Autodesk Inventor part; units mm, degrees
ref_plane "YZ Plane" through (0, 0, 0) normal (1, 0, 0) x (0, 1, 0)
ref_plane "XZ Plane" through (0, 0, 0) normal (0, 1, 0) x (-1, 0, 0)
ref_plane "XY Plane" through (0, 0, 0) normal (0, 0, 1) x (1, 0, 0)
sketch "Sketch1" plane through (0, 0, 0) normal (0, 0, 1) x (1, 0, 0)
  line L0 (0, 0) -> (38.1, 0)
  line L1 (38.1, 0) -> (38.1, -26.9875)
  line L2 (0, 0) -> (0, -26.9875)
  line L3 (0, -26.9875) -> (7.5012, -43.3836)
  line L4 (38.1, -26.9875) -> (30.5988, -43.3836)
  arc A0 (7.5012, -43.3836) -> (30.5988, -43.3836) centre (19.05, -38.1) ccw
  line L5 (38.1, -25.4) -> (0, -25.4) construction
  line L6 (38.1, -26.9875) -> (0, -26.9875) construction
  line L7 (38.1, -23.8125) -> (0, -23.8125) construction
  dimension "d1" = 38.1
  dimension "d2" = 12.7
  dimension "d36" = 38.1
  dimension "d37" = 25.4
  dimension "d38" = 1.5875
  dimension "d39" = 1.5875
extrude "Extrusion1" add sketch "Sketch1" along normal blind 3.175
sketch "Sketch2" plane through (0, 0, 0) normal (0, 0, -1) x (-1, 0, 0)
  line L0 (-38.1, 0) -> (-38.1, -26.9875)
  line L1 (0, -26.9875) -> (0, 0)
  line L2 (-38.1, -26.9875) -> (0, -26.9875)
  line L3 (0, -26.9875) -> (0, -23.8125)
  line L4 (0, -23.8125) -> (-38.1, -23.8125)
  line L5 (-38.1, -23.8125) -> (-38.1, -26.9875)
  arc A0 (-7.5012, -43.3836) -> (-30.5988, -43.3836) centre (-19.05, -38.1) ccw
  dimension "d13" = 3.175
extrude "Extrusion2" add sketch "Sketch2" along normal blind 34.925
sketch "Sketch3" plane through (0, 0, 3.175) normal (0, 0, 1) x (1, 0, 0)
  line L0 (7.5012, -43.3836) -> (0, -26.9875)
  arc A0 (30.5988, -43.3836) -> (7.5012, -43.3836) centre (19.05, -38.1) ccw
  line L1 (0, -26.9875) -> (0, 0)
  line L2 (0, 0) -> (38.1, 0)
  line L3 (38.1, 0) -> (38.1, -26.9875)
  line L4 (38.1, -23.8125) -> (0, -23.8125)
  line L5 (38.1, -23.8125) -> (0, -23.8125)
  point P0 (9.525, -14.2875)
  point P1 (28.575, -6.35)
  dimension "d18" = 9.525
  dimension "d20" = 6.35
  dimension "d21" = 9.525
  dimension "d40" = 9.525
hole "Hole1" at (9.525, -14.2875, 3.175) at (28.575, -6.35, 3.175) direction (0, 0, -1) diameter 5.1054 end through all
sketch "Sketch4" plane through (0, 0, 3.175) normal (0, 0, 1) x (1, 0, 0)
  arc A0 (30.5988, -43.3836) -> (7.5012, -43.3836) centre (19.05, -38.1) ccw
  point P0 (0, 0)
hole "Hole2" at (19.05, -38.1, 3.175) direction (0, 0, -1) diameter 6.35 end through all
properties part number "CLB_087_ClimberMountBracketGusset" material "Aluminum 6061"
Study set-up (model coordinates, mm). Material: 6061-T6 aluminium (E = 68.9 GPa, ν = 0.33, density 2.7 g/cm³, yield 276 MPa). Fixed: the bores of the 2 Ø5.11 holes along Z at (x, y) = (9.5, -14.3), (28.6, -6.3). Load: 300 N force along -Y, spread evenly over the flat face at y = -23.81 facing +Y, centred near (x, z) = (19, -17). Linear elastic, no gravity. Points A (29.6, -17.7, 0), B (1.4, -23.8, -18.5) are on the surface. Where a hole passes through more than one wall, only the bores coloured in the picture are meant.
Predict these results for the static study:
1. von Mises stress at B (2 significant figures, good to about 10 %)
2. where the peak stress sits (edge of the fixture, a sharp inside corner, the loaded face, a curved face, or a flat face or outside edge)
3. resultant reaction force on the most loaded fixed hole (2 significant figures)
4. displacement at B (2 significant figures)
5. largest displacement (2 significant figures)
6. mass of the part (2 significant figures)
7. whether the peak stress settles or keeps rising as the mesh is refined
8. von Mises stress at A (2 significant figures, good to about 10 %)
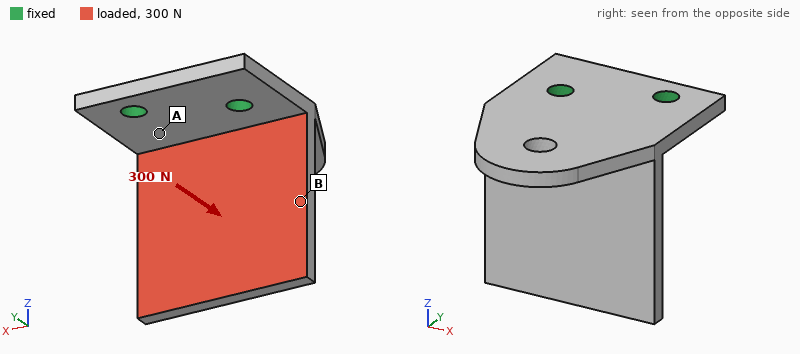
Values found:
20 MPa
edge of the fixture
170 N
0.27 mm
0.58 mm
25 g
keeps rising
63 MPa
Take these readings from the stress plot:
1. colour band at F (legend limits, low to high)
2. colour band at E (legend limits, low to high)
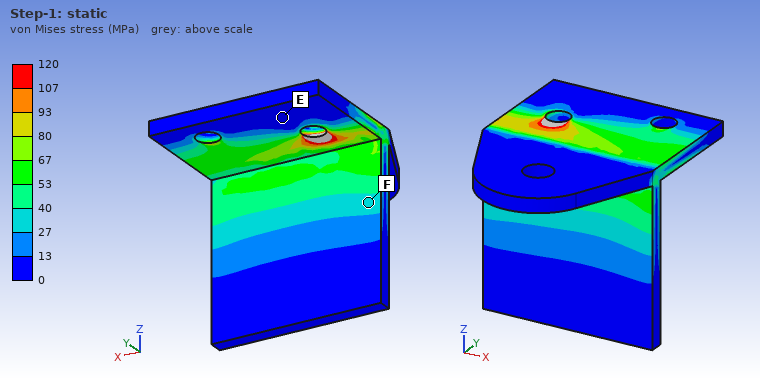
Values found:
27 to 40 MPa
0 to 13 MPa
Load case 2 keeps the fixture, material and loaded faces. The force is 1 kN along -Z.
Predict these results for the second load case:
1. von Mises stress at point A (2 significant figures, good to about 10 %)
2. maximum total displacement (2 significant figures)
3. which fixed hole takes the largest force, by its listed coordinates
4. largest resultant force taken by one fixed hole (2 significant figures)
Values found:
48 MPa
0.32 mm
(9.5, -14.3)
710 N
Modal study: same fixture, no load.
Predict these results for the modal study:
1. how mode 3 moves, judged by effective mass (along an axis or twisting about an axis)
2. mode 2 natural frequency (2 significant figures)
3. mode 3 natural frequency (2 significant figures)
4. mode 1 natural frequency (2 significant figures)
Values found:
along Z
2600 Hz
3700 Hz
1200 Hz
